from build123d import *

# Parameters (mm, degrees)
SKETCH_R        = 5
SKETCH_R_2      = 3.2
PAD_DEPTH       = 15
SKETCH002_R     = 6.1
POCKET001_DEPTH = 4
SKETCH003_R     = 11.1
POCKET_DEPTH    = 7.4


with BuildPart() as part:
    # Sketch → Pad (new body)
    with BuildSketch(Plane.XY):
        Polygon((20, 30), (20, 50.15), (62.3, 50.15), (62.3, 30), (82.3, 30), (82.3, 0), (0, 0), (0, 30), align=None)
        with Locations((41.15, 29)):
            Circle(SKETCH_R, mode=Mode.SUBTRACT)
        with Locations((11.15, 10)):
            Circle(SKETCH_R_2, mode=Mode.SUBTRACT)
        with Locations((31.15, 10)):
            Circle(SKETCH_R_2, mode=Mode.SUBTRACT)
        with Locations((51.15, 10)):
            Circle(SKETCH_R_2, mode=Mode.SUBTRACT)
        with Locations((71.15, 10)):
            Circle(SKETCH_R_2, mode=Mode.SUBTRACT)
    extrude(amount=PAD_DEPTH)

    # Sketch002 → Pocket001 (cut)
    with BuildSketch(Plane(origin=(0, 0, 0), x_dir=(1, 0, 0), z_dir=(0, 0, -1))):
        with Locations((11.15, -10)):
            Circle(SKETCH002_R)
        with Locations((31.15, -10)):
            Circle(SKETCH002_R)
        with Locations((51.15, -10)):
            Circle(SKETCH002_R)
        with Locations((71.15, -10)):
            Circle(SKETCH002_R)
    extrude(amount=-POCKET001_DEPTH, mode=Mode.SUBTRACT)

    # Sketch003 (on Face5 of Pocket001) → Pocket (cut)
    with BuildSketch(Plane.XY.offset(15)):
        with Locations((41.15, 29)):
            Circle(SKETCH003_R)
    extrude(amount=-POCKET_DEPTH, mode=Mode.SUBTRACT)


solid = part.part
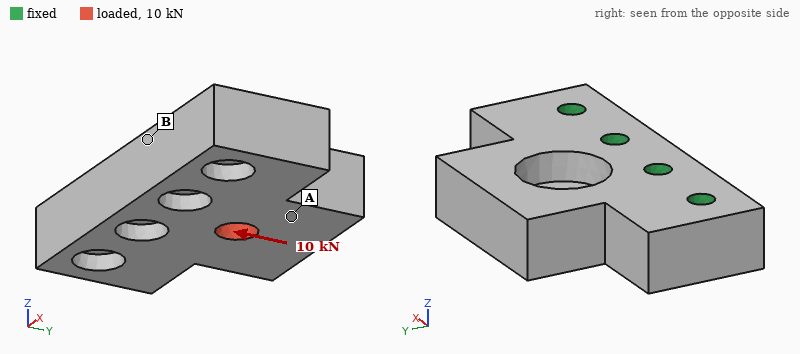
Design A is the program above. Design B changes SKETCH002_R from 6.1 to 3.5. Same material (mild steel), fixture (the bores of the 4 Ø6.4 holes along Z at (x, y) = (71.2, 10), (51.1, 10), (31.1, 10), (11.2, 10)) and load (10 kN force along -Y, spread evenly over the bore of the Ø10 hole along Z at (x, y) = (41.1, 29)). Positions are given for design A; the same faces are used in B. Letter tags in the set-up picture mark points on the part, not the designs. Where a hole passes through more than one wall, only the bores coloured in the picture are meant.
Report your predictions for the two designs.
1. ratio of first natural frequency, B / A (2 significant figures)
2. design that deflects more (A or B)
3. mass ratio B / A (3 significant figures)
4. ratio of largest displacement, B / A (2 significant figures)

1.0
A
1.03
0.85
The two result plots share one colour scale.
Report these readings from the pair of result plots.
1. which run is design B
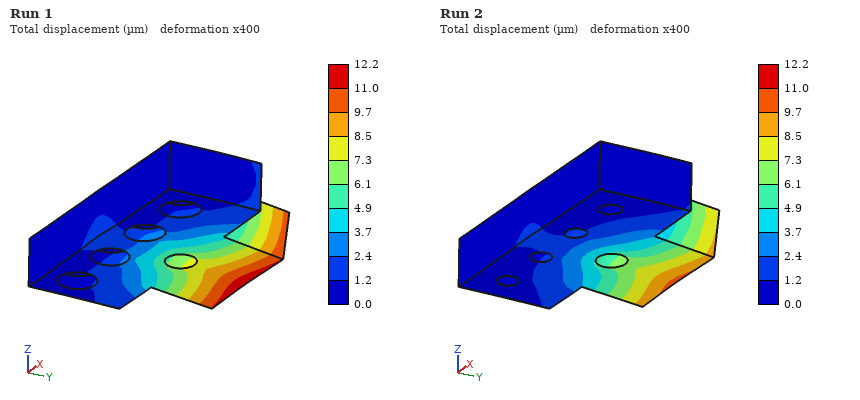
Run 2
